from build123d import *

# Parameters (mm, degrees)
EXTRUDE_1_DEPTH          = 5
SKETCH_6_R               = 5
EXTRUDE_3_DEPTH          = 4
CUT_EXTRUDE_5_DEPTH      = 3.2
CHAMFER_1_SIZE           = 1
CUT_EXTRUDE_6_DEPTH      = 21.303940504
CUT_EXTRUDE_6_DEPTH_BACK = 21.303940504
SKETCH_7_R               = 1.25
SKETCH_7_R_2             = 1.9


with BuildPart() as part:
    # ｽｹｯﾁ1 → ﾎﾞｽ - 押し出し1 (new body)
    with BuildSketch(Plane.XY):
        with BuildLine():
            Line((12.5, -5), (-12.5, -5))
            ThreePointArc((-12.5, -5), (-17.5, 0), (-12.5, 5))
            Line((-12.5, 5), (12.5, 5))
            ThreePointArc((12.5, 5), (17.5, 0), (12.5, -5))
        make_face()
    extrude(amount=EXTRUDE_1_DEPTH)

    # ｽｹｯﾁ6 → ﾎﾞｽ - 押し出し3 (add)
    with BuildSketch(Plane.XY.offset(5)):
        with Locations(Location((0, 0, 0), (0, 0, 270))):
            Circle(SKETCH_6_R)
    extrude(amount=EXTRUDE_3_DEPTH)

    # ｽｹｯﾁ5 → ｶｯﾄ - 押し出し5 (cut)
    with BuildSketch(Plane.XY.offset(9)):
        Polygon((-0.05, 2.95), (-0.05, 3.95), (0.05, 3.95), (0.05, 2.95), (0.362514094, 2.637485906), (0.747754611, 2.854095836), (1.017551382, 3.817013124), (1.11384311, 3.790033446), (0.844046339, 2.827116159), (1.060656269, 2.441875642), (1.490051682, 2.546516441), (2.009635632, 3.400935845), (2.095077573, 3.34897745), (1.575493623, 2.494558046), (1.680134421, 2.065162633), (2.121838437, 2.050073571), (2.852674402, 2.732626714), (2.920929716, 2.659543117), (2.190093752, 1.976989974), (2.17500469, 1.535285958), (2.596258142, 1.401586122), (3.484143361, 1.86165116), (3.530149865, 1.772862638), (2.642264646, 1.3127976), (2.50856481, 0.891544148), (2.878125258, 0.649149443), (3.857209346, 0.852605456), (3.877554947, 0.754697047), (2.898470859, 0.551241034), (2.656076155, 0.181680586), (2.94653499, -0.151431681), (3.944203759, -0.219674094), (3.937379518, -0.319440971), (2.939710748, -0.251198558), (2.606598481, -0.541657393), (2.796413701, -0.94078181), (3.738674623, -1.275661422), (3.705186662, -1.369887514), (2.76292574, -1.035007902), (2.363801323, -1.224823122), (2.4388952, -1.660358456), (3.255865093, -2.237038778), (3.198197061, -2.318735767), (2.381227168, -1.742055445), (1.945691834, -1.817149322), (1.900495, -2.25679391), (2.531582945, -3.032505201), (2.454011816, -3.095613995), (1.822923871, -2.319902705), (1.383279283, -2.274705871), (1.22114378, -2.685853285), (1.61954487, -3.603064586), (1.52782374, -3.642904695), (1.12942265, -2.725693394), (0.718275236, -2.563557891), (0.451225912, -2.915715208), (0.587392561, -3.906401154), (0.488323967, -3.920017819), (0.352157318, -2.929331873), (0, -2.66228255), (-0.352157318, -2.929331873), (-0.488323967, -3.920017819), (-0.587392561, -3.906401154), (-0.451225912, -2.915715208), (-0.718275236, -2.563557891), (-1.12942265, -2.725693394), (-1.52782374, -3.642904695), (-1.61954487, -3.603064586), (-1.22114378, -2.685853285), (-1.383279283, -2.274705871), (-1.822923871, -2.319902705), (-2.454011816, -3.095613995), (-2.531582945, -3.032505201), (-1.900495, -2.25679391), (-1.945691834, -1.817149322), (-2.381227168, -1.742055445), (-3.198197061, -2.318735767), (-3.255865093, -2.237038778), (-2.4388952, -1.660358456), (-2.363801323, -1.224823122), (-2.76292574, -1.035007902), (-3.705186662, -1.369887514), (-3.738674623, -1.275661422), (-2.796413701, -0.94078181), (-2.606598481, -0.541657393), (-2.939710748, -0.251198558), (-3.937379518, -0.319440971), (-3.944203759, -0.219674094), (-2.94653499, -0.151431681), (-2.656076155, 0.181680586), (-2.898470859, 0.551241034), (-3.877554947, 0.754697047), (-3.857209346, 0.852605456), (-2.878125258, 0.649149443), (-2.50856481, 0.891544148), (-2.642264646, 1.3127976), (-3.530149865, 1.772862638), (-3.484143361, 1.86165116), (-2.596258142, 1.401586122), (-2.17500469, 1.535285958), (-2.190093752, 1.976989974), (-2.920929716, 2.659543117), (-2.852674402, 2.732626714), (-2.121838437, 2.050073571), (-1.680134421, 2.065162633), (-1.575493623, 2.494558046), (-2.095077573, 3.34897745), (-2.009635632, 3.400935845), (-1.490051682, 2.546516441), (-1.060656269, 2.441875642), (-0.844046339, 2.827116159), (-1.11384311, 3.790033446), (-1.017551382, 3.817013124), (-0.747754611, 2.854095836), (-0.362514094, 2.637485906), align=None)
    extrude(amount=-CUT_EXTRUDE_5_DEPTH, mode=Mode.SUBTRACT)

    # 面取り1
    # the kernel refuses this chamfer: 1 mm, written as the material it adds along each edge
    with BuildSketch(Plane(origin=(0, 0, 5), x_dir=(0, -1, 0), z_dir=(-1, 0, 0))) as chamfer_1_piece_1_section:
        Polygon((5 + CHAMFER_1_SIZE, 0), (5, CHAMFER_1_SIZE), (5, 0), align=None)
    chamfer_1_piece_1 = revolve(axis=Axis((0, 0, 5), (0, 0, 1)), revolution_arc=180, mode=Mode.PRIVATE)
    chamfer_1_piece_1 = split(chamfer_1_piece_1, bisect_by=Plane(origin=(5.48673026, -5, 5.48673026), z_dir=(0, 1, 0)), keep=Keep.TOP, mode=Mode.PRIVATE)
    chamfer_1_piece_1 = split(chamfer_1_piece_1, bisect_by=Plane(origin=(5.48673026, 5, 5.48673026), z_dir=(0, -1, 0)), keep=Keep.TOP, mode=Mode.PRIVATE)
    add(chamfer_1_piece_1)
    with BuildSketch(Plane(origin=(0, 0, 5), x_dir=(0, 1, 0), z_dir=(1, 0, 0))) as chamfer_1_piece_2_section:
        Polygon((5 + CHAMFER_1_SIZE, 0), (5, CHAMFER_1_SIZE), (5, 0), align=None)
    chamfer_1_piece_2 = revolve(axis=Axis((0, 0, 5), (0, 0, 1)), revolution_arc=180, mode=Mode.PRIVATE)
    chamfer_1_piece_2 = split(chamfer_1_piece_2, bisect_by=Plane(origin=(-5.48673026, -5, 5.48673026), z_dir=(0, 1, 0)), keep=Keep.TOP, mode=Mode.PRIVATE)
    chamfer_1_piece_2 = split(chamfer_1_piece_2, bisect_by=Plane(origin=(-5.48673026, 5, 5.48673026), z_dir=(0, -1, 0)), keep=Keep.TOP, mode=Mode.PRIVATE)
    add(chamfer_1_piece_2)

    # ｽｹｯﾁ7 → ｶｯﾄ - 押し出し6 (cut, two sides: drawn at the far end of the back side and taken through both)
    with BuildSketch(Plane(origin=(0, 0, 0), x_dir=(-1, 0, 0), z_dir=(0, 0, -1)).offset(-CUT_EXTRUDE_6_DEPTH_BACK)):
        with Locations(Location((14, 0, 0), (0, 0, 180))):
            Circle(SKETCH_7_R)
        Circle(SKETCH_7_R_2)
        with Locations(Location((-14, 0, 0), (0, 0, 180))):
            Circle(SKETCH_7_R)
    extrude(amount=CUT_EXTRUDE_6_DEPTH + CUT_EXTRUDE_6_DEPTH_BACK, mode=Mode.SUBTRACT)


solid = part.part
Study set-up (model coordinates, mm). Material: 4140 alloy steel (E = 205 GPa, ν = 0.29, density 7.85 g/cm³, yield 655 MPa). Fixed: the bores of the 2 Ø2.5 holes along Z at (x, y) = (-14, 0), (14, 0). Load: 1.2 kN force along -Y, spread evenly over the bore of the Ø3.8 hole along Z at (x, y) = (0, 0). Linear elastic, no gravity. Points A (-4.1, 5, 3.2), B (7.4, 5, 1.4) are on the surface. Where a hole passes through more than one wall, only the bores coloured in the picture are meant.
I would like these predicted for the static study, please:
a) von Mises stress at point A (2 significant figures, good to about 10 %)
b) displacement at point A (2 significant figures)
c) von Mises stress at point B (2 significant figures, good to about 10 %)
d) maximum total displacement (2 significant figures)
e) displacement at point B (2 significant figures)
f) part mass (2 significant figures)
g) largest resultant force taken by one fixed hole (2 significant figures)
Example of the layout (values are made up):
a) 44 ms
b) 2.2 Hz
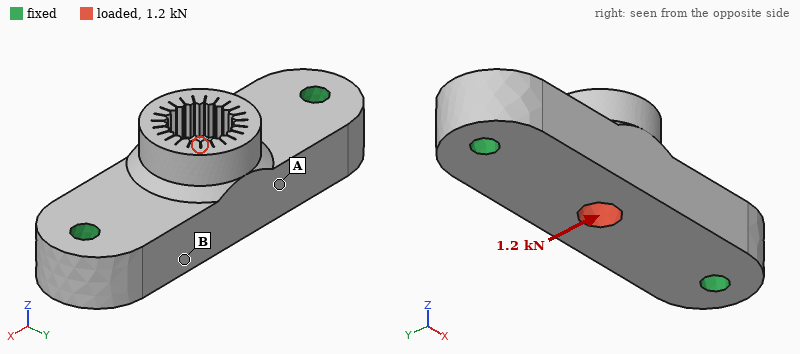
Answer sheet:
a) 42 MPa
b) 4.4 µm
c) 17 MPa
d) 5.5 µm
e) 3.2 µm
f) 14 g
g) 600 N
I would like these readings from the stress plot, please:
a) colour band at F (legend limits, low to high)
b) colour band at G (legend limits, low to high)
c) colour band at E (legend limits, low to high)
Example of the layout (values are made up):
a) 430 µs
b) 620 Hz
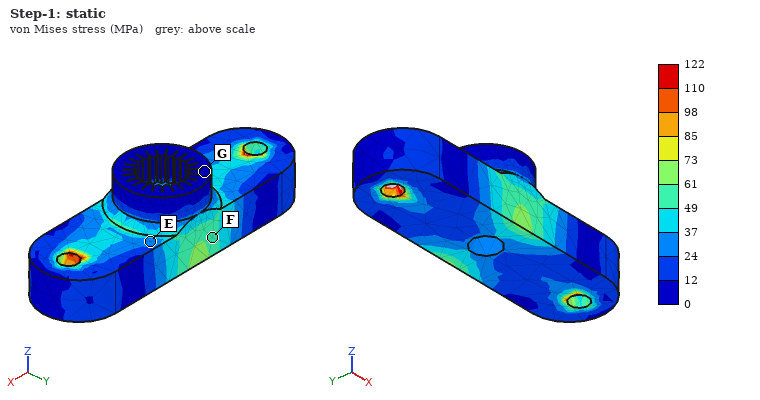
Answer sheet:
a) 49 to 61 MPa
b) 0 to 12 MPa
c) 24 to 37 MPa
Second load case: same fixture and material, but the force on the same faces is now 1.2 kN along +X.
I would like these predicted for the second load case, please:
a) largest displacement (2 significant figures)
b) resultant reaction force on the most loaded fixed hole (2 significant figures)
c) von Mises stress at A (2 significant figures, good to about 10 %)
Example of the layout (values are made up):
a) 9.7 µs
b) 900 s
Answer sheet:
a) 0.98 µm
b) 600 N
c) 7.1 MPa
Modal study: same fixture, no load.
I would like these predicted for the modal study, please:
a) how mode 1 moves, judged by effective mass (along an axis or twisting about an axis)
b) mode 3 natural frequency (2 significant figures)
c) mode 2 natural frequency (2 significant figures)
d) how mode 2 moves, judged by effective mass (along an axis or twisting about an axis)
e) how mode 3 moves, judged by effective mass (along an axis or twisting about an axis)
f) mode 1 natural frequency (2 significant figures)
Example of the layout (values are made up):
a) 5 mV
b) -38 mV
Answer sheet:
a) along Z
b) 37 kHz
c) 27 kHz
d) along Y
e) along Y
f) 26 kHz
